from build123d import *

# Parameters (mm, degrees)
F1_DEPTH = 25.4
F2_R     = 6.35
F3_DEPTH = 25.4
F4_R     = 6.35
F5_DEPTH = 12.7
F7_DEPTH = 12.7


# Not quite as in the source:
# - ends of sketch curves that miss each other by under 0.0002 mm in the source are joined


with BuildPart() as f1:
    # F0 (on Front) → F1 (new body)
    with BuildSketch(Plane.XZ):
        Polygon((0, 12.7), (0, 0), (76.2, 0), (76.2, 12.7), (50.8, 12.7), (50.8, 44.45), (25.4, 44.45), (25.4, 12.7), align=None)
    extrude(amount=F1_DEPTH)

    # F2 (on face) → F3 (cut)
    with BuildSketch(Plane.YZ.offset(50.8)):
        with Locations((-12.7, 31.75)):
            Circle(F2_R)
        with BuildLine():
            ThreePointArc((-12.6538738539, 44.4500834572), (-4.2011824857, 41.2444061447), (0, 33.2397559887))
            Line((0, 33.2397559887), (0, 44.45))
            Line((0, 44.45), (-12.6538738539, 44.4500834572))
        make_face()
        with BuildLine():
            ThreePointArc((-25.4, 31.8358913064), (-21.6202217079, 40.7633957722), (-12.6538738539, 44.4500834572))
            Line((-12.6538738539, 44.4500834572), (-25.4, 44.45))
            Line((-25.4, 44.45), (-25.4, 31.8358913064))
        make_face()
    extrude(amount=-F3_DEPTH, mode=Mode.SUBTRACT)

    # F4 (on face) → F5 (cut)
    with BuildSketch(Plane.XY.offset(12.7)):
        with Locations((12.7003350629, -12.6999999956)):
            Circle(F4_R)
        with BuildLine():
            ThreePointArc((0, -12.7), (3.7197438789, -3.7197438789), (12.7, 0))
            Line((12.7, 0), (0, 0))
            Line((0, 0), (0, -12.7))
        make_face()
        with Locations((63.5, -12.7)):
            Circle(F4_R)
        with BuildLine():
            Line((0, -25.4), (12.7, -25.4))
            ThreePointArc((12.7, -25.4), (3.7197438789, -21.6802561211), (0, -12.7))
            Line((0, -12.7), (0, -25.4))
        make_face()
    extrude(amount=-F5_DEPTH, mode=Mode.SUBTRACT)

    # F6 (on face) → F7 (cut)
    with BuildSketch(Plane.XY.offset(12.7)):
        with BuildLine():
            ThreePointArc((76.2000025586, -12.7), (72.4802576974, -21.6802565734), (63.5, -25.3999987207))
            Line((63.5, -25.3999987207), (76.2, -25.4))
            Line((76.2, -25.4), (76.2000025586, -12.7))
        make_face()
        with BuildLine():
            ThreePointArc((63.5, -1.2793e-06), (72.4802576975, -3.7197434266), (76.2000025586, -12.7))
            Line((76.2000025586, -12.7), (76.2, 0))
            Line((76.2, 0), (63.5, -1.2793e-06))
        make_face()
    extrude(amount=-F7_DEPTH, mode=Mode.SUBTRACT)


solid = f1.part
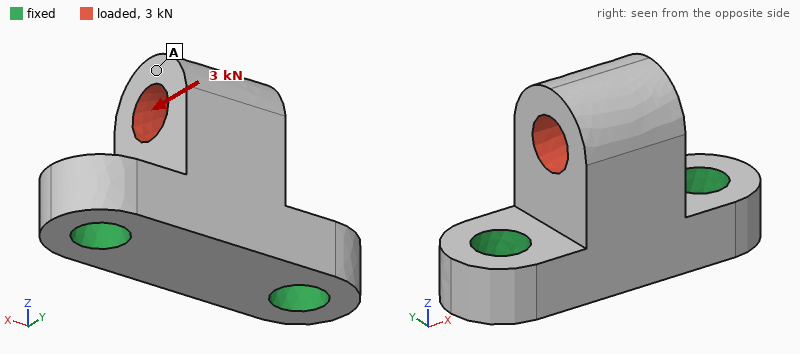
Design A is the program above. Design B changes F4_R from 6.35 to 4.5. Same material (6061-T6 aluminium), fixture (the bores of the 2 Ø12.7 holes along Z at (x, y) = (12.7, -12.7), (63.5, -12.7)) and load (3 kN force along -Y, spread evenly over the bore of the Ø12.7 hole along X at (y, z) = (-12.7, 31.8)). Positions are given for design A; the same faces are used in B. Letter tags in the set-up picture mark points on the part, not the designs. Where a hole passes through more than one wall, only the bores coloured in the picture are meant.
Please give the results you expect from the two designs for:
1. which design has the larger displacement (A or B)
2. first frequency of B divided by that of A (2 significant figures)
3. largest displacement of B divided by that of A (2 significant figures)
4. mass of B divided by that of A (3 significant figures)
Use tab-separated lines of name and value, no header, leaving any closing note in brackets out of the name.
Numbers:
which design has the larger displacement	B
first frequency of B divided by that of A	0.90
largest displacement of B divided by that of A	1.2
mass of B divided by that of A	1.05
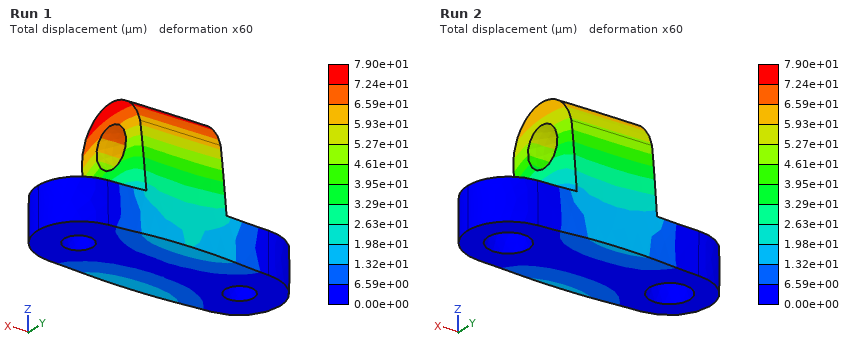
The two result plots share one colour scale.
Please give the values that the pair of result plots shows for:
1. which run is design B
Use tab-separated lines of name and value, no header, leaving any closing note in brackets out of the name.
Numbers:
which run is design B	Run 1
